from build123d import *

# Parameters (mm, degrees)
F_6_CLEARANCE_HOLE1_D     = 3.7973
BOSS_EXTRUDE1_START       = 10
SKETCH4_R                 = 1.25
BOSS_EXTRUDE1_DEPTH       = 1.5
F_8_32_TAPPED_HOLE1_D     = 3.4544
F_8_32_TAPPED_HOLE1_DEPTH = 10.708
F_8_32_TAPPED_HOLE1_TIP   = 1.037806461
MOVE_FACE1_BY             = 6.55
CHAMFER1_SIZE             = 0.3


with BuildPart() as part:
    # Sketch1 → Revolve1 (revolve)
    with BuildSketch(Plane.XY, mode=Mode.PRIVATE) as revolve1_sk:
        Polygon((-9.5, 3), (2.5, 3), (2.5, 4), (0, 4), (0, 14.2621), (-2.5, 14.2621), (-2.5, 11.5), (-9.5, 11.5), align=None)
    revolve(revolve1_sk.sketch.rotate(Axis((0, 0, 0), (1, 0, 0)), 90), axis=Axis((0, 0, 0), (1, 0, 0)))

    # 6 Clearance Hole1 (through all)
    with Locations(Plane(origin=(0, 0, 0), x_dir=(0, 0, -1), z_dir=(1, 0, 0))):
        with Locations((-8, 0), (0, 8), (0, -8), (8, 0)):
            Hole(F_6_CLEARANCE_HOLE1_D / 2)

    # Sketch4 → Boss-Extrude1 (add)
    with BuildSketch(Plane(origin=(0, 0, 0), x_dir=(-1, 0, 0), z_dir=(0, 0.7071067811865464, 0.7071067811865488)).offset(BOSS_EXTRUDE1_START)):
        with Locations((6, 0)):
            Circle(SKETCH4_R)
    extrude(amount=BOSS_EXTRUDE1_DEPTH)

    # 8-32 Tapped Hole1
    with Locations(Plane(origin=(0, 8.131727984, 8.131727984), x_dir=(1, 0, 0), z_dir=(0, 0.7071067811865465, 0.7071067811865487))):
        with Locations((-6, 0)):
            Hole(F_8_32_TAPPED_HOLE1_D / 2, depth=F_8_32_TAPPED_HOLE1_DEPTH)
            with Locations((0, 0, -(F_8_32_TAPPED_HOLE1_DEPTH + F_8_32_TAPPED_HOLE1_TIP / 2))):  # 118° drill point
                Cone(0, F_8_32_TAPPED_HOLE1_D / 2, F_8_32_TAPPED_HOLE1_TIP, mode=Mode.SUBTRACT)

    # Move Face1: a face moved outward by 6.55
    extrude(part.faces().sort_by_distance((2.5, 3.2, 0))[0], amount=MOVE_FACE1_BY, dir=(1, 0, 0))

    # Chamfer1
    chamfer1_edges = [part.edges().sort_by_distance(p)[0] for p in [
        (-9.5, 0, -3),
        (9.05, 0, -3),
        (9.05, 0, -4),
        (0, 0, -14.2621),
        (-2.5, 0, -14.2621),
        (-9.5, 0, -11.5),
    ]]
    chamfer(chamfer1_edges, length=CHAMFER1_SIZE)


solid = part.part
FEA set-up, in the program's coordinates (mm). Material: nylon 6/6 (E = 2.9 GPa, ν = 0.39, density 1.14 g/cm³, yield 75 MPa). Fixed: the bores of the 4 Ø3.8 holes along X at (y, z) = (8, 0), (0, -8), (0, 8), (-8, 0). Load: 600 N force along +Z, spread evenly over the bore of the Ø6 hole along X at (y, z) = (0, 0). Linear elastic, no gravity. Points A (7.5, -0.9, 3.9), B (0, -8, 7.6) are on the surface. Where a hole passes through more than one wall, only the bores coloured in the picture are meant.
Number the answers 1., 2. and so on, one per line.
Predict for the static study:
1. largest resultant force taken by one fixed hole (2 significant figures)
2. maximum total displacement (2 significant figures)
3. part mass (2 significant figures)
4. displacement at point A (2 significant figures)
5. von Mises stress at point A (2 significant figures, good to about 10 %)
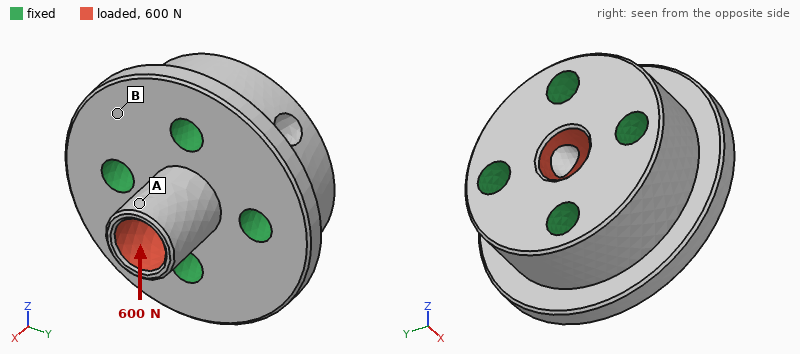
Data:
1. 270 N
2. 0.23 mm
3. 4.5 g
4. 0.21 mm
5. 6.1 MPa
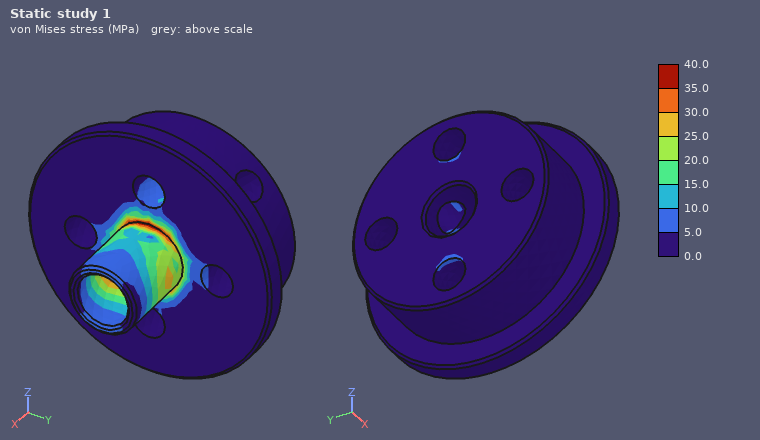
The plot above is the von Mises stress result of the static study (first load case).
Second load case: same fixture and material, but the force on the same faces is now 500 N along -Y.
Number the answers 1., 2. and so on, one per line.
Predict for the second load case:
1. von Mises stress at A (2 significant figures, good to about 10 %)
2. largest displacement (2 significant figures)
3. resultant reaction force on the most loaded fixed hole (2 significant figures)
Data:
1. 5.5 MPa
2. 0.19 mm
3. 220 N
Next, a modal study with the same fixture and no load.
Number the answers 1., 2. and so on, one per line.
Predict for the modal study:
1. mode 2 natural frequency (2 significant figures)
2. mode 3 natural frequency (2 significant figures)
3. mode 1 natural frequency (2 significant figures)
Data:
1. 14 kHz
2. 19 kHz
3. 14 kHz
